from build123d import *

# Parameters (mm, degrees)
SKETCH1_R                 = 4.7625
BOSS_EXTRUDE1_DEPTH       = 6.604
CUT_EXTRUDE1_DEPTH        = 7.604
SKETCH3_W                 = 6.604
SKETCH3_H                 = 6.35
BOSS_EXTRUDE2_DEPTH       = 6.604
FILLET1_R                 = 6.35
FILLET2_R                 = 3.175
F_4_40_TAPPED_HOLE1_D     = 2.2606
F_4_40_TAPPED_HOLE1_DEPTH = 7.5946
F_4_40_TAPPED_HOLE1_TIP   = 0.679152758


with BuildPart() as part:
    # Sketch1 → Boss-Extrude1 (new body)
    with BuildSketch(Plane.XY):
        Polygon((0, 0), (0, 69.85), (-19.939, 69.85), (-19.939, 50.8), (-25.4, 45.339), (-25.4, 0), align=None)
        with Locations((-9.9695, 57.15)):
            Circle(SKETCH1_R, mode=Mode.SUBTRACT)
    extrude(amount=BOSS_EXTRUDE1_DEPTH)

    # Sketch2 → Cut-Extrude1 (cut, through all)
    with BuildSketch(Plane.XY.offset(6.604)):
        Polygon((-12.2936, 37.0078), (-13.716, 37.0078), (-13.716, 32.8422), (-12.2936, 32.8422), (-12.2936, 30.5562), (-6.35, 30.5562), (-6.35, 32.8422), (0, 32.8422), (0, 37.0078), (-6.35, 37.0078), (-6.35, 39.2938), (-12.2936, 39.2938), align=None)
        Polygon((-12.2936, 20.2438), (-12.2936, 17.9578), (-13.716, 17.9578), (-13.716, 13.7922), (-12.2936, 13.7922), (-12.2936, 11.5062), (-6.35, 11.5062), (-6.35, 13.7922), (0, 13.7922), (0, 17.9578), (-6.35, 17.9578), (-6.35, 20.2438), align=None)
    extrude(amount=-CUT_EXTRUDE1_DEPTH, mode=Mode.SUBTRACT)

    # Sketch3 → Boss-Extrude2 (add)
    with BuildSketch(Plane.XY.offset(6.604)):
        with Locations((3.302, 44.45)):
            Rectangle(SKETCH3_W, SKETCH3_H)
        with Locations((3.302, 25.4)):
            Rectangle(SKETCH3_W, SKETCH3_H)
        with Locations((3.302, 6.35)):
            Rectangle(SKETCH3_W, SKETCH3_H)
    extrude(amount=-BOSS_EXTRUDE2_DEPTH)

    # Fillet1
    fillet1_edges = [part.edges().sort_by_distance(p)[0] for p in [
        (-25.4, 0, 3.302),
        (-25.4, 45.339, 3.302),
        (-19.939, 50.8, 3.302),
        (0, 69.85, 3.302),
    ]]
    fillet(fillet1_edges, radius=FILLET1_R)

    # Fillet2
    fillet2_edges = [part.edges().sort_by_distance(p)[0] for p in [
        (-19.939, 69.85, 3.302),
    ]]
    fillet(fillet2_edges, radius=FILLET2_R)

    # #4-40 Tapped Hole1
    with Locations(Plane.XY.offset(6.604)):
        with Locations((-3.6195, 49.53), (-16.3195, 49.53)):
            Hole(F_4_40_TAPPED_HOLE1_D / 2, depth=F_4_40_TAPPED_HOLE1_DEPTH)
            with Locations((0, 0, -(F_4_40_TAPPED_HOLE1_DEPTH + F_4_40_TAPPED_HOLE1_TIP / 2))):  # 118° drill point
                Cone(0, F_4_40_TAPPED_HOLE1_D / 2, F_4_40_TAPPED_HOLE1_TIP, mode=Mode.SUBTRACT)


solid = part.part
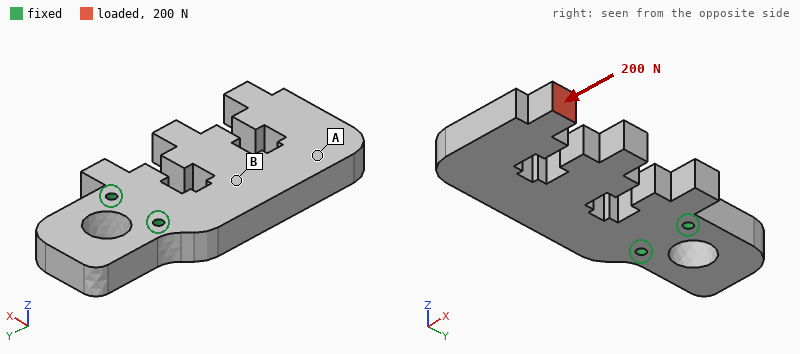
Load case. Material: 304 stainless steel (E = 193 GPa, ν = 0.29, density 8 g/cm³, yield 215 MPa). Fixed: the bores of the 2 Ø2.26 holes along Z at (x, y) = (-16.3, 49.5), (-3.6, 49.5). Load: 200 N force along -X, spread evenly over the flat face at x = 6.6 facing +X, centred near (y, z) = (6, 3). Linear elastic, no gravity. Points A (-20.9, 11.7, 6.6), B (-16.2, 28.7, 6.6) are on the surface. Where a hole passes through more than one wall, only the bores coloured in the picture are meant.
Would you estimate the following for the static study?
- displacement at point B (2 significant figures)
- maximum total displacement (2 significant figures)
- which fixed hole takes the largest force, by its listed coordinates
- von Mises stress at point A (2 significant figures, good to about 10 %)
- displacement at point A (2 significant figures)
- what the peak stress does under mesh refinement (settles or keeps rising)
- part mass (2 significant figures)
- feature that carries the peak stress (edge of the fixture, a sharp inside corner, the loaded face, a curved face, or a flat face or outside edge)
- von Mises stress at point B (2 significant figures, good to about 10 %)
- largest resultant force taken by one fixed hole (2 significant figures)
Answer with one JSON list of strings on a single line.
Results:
["7.4 µm", "36 µm", "(-3.6, 49.5)", "6.2 MPa", "21 µm", "keeps rising", "80 g", "edge of the fixture", "14 MPa", "710 N"]
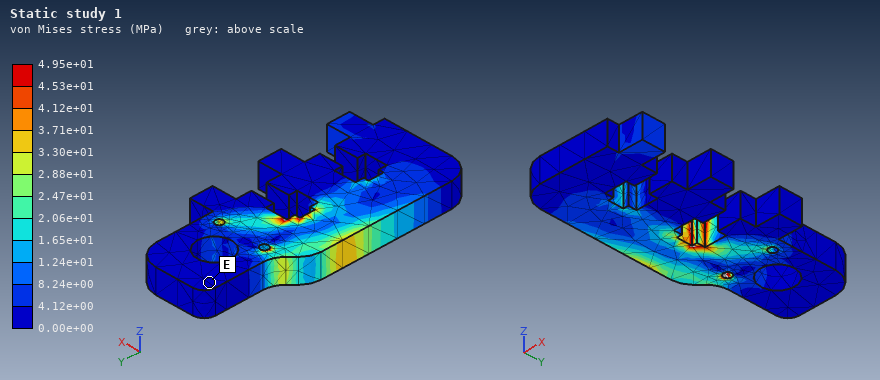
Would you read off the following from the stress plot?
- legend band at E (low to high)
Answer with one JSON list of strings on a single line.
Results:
["0.00e+00 to 4.12e+00 MPa"]
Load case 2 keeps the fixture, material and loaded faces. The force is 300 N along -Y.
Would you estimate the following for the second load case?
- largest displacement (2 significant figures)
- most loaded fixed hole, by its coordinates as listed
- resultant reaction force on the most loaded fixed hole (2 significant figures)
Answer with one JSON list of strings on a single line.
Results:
["62 µm", "(-3.6, 49.5)", "570 N"]
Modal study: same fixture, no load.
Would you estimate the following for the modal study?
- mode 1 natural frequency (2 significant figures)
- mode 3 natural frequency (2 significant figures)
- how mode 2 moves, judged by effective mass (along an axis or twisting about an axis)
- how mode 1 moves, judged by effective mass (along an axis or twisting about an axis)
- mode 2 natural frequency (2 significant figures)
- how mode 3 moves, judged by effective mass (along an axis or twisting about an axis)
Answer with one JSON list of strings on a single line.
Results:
["1400 Hz", "4100 Hz", "along X", "along Z", "2600 Hz", "twisting about Y"]
